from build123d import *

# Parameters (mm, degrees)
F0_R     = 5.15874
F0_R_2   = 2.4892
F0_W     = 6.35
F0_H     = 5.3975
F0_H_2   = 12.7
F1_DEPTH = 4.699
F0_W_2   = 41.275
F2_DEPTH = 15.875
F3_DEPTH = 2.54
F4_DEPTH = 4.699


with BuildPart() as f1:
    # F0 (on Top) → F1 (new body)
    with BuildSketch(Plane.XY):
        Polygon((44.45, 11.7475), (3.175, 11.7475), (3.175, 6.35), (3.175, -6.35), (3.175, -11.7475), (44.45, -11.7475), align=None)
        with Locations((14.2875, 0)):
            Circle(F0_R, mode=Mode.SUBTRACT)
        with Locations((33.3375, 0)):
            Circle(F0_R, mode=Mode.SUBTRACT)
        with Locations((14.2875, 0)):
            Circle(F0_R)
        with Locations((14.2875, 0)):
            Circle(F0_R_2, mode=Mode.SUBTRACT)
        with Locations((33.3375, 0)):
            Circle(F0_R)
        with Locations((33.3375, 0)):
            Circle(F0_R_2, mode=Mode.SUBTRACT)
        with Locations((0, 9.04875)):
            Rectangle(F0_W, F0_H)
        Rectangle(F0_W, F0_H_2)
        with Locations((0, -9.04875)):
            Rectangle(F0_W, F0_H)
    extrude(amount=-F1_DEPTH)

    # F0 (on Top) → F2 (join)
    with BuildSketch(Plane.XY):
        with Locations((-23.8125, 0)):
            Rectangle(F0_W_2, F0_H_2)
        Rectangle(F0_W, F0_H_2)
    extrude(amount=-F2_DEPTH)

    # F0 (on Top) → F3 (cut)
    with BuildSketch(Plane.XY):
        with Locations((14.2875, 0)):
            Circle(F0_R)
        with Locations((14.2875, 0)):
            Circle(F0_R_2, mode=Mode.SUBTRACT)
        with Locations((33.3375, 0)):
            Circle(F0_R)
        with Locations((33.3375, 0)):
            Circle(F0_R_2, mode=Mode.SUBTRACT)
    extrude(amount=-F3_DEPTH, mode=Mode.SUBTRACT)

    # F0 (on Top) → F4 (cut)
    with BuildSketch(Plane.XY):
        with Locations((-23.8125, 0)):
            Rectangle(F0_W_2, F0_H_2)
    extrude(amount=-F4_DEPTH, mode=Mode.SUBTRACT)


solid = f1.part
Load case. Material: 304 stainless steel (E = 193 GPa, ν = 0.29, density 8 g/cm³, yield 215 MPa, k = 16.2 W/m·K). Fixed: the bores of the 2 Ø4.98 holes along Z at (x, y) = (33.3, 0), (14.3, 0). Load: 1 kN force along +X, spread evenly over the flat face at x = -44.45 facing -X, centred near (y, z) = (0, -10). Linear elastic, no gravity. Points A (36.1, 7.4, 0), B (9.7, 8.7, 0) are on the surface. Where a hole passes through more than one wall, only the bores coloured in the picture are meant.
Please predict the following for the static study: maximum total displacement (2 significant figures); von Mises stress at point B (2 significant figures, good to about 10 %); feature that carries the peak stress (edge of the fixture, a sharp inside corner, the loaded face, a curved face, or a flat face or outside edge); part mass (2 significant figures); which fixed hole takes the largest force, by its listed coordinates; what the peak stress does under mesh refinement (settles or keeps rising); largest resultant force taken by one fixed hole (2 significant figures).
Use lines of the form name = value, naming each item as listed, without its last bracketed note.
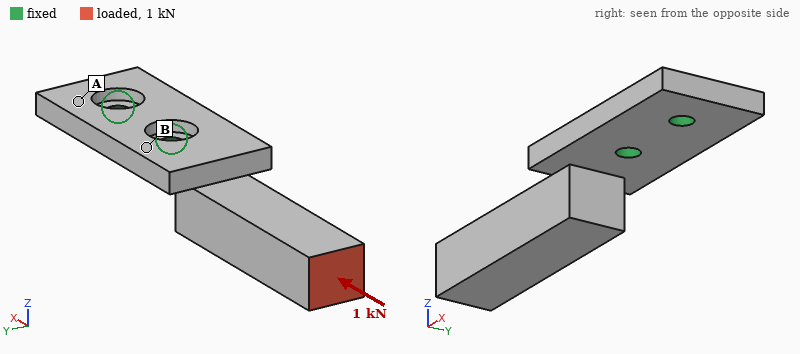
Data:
maximum total displacement = 0.21 mm
von Mises stress at point B = 100 MPa
feature that carries the peak stress = edge of the fixture
part mass = 92 g
which fixed hole takes the largest force, by its listed coordinates = (14.3, 0)
what the peak stress does under mesh refinement = keeps rising
largest resultant force taken by one fixed hole = 1.4 kN
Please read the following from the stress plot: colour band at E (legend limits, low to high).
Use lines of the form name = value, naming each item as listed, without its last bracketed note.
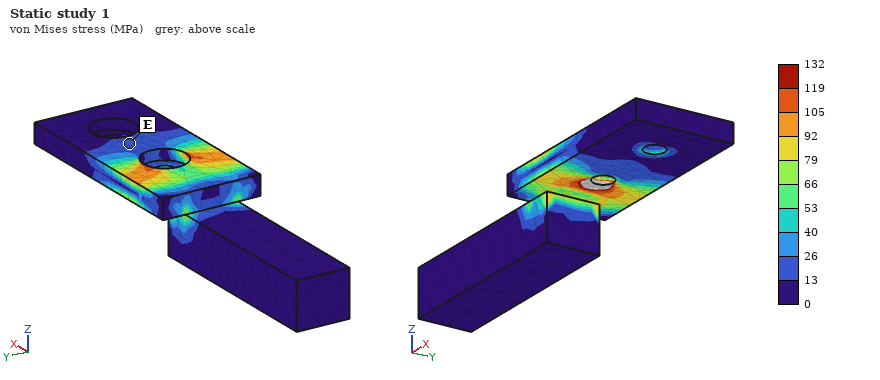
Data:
colour band at E = 13 to 26 MPa
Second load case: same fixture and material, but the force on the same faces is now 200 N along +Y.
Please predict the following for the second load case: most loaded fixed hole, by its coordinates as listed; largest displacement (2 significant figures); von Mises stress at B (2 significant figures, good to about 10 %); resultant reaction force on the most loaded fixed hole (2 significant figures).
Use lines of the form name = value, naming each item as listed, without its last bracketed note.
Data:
most loaded fixed hole, by its coordinates as listed = (14.3, 0)
largest displacement = 55 µm
von Mises stress at B = 18 MPa
resultant reaction force on the most loaded fixed hole = 680 N
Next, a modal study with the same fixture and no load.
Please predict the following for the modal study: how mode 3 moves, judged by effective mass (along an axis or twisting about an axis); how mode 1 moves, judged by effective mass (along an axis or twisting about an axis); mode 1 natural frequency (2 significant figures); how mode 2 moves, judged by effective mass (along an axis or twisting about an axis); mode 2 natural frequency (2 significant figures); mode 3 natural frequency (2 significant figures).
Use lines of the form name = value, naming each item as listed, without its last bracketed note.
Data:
how mode 3 moves, judged by effective mass = twisting about X
how mode 1 moves, judged by effective mass = along Z
mode 1 natural frequency = 860 Hz
how mode 2 moves, judged by effective mass = along Y
mode 2 natural frequency = 2300 Hz
mode 3 natural frequency = 5000 Hz
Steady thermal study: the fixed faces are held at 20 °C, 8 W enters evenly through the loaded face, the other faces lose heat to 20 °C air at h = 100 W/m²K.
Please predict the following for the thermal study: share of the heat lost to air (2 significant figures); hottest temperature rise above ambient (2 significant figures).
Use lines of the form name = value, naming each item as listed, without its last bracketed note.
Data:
share of the heat lost to air = 94 %
hottest temperature rise above ambient = 77 K
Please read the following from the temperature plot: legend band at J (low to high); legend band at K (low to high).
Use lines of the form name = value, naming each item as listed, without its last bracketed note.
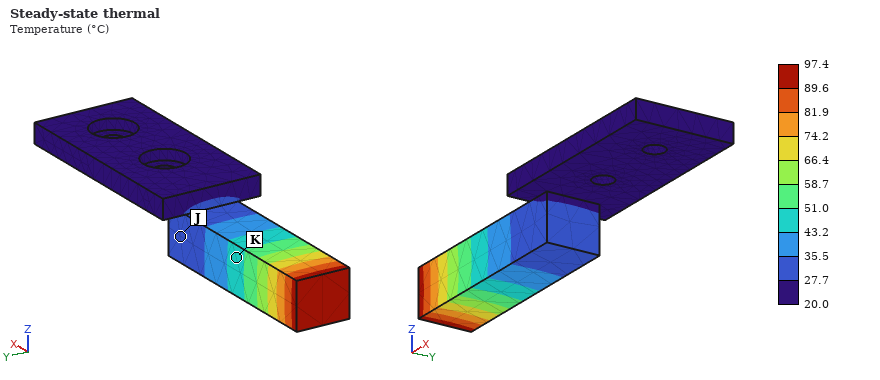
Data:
legend band at J = 27.7 to 35.5 °C
legend band at K = 43.2 to 51.0 °C
